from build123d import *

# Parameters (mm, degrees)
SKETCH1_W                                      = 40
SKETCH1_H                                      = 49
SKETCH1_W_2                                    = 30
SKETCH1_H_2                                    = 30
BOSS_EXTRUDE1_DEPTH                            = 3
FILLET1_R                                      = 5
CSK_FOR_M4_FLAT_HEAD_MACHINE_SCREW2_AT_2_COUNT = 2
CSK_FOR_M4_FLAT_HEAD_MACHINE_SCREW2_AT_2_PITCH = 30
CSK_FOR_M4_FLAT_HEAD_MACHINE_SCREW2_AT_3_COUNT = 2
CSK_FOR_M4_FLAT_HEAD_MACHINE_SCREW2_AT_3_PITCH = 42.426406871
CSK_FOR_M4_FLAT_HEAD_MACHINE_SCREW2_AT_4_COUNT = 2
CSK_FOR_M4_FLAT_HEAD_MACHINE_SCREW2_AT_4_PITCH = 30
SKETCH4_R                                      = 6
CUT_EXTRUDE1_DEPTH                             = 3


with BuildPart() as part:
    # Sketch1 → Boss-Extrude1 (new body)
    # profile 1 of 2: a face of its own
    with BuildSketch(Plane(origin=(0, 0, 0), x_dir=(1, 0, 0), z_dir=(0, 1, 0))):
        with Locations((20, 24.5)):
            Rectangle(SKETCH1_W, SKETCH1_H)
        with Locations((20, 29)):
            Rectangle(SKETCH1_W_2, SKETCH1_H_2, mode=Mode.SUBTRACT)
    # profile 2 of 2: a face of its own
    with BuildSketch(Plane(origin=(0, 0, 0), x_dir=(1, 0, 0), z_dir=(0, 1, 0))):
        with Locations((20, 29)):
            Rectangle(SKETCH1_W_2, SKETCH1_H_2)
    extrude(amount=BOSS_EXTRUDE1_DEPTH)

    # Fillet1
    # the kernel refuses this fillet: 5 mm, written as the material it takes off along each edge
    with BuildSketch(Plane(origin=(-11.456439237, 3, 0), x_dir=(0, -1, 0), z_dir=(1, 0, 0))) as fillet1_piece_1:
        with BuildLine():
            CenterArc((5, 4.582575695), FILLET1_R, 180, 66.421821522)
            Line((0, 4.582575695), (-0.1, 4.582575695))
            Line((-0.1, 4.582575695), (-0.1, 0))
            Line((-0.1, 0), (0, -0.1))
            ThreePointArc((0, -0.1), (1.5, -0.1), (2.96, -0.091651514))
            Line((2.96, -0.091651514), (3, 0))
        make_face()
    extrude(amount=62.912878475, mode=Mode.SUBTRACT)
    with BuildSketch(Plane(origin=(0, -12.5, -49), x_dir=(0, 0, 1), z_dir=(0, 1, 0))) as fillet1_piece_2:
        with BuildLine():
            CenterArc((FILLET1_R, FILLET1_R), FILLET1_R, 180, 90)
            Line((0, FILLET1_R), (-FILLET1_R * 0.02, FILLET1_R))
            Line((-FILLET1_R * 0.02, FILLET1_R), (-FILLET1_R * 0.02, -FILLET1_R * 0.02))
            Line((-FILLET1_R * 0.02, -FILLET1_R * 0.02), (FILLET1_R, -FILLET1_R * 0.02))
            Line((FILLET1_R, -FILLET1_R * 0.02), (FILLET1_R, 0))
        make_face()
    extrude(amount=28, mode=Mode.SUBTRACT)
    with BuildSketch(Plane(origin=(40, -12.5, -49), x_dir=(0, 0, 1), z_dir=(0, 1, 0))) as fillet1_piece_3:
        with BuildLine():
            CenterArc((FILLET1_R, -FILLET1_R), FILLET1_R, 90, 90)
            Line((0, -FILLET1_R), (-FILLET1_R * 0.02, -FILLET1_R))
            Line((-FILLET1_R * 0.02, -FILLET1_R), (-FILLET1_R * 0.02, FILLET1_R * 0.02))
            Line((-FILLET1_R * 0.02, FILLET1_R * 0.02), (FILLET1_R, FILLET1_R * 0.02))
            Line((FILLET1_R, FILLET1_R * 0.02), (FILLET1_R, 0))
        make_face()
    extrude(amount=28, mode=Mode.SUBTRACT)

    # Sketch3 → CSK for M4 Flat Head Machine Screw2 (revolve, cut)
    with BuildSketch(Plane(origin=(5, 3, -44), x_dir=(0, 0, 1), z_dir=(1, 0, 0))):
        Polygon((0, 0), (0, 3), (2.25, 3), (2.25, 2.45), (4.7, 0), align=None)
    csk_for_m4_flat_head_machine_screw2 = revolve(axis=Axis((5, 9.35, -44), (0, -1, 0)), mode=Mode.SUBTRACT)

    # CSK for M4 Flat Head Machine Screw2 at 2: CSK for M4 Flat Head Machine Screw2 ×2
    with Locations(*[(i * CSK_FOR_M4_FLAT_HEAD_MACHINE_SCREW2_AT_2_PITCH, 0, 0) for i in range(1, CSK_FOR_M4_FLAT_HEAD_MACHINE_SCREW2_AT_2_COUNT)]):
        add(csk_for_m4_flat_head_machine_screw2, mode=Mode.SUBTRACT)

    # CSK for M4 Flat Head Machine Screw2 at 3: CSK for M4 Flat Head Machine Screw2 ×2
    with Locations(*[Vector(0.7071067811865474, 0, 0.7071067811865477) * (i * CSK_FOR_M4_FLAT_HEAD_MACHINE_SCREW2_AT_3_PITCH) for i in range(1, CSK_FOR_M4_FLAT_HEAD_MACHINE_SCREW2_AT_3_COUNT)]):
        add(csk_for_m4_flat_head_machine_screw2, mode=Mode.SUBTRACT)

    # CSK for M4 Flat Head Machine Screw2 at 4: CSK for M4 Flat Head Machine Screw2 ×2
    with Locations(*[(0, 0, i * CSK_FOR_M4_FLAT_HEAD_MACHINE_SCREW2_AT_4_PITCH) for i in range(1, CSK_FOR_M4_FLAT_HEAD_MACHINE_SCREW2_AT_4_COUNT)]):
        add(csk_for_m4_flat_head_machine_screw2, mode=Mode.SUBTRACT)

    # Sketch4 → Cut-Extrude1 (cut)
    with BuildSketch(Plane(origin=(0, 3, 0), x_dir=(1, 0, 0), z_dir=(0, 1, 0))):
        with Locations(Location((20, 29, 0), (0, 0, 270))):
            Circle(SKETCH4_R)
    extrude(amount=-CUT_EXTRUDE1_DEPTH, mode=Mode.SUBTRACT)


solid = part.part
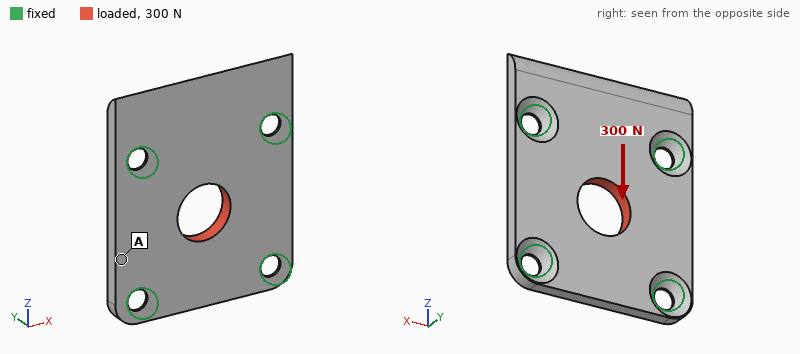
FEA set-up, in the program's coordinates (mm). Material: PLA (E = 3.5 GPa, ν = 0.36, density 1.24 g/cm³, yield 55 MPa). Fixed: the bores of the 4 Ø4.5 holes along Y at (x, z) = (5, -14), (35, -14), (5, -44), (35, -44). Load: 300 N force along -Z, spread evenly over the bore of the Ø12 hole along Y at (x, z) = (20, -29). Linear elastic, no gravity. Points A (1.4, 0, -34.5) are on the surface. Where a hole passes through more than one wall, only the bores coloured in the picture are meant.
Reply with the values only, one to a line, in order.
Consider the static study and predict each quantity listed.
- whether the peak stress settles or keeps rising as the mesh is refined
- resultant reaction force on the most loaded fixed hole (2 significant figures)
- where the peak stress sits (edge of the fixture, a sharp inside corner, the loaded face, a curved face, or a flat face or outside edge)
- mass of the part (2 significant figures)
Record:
keeps rising
81 N
edge of the fixture
6.1 g
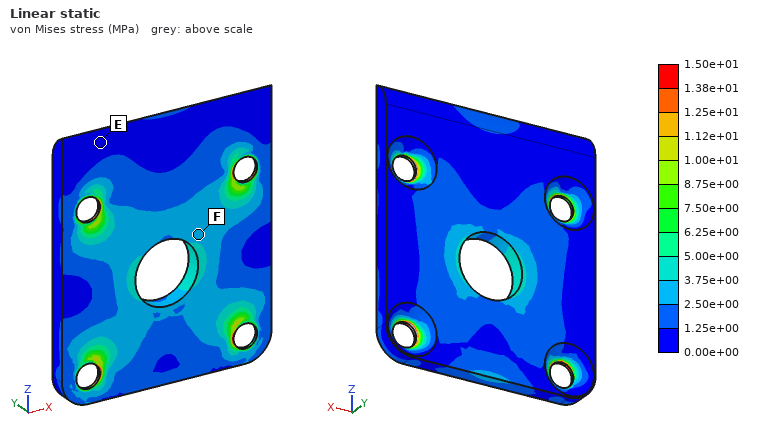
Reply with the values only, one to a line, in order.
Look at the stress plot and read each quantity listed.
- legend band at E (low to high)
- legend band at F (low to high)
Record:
0.00e+00 to 1.25e+00 MPa
2.50e+00 to 3.75e+00 MPa
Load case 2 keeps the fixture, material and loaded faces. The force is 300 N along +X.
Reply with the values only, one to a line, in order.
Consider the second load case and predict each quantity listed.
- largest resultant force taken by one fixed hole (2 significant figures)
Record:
80 N
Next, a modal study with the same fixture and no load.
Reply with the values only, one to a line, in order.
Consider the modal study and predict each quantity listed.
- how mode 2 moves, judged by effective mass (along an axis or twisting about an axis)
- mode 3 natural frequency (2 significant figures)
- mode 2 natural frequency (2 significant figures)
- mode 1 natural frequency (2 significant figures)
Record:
along Y
4300 Hz
3600 Hz
2700 Hz
